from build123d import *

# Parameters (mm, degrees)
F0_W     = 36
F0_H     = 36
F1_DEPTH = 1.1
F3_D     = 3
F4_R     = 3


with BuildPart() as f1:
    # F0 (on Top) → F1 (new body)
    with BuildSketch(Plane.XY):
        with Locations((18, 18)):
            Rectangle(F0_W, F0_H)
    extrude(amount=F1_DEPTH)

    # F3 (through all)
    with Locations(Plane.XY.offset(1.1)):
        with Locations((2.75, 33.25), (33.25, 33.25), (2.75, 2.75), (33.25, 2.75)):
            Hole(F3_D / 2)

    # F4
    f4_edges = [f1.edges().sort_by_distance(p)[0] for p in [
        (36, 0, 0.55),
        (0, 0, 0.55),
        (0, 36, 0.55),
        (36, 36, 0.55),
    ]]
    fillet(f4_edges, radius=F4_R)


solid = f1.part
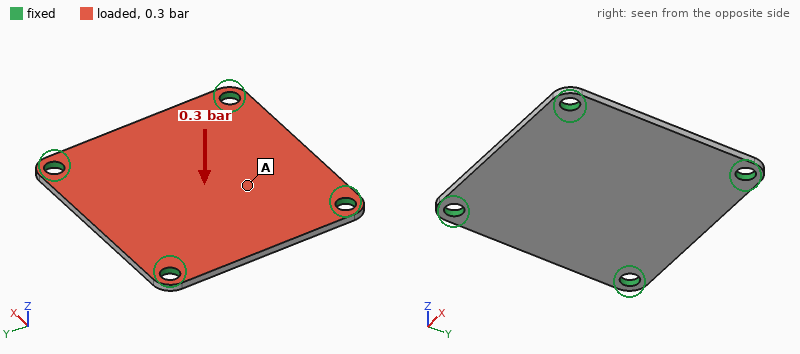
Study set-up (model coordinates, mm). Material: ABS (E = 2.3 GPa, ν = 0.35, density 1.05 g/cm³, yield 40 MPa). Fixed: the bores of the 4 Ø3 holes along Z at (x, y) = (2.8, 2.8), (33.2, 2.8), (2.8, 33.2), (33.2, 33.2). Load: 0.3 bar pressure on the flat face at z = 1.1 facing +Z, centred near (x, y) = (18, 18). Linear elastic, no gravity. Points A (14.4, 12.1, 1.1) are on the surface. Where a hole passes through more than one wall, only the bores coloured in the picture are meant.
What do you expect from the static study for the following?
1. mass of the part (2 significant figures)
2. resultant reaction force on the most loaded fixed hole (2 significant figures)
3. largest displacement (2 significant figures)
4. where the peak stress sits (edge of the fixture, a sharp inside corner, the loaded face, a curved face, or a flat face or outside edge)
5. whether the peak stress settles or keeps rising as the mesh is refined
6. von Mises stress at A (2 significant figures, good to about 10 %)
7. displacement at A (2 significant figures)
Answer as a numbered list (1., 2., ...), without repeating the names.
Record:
1. 1.5 g
2. 9.5 N
3. 0.55 mm
4. edge of the fixture
5. keeps rising
6. 5.7 MPa
7. 0.47 mm
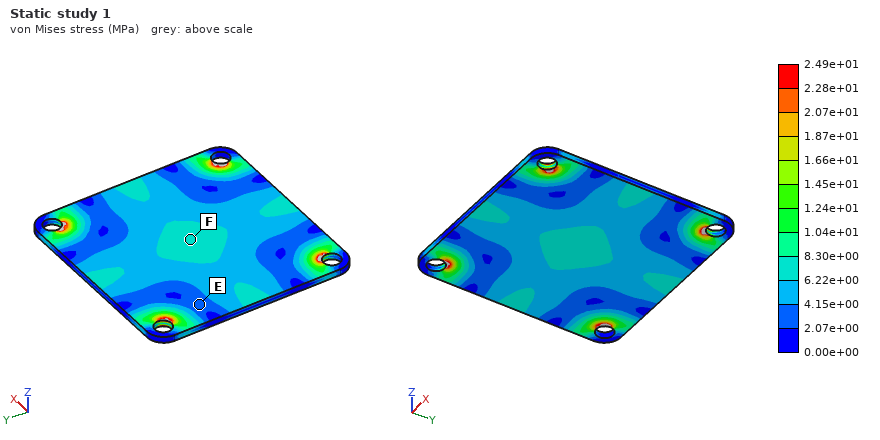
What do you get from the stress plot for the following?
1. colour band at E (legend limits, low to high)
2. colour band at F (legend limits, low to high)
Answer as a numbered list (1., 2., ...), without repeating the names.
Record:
1. 2.07e+00 to 4.15e+00 MPa
2. 6.22e+00 to 8.30e+00 MPa
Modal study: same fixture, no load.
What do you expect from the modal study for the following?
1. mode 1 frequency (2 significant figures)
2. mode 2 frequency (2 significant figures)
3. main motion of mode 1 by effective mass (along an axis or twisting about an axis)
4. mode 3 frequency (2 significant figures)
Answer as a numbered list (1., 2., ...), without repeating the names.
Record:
1. 1300 Hz
2. 2200 Hz
3. along Z
4. 2200 Hz
